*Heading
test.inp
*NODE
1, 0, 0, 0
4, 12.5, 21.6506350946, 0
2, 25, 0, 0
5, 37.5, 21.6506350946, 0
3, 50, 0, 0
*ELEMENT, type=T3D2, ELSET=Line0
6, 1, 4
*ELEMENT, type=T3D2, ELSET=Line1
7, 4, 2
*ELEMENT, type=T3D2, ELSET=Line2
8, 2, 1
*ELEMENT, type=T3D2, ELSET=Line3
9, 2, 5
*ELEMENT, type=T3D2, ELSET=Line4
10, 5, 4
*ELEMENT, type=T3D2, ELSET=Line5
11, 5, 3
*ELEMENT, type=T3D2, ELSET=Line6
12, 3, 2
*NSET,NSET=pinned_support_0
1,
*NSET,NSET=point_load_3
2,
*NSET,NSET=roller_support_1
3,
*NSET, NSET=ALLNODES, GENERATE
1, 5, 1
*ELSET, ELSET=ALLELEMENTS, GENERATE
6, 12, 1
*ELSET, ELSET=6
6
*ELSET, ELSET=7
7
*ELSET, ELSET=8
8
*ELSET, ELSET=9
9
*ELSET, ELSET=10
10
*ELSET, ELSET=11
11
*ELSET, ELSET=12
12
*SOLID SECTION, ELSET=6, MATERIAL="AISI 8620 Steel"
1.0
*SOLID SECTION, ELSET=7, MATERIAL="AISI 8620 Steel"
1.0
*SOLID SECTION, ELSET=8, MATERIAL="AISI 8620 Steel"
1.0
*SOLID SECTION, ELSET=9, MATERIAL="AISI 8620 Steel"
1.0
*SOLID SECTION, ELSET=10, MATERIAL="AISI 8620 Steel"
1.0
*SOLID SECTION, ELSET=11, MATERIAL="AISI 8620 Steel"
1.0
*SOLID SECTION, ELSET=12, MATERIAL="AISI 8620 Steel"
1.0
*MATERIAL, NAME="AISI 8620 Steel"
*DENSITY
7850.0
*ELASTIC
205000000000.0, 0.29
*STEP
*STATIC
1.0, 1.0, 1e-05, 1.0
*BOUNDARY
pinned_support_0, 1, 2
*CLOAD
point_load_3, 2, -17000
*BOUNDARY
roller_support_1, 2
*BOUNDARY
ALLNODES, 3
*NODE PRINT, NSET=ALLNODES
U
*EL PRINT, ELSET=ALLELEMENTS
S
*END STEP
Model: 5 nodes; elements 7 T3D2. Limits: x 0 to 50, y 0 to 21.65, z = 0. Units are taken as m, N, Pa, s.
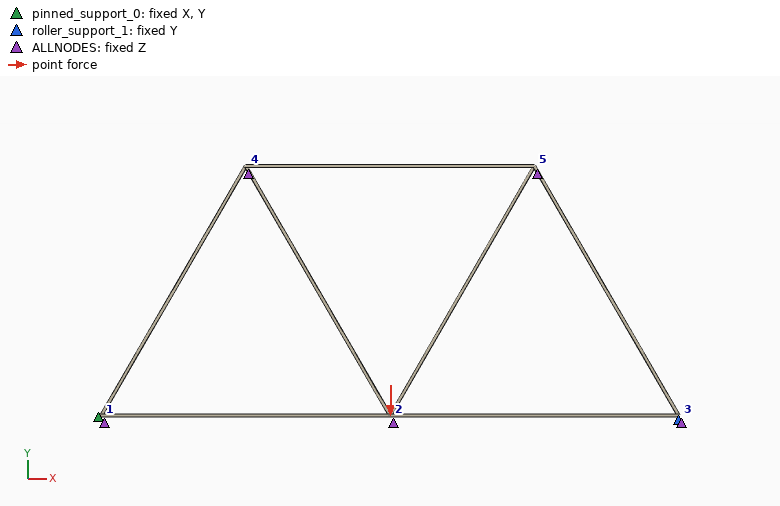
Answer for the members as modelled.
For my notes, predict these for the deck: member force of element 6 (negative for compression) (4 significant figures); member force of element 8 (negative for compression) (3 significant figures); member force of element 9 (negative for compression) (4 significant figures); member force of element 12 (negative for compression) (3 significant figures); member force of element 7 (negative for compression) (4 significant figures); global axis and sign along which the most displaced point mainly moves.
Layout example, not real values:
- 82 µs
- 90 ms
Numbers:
- -9815 N
- 4910 N
- 9815 N
- 4910 N
- 9815 N
- -Y
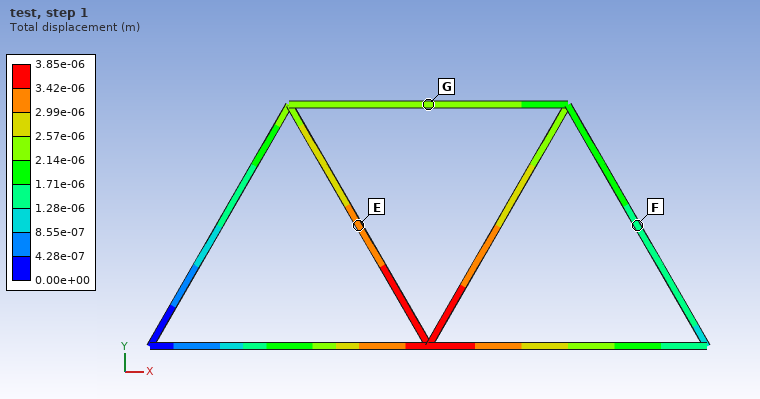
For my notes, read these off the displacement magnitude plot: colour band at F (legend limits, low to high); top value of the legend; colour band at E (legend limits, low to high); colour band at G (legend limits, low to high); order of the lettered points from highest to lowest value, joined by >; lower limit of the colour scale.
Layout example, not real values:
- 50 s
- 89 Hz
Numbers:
- 1.28e-06 to 1.71e-06 m
- 3.85e-06 m
- 2.99e-06 to 3.42e-06 m
- 2.14e-06 to 2.57e-06 m
- E > G > F
- 0.00e+00 m
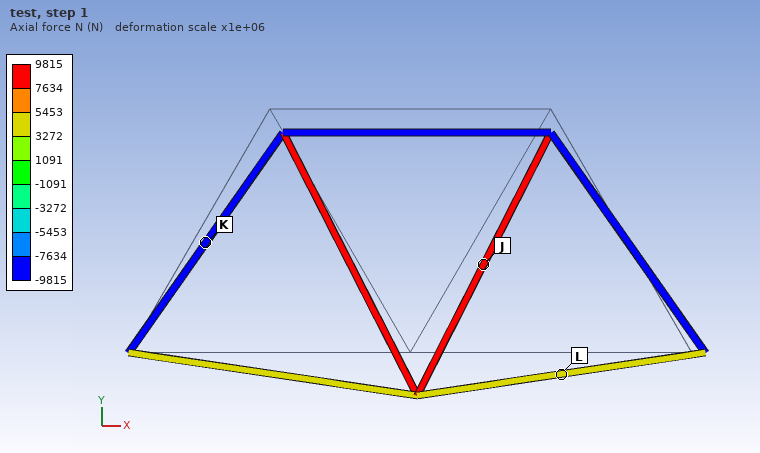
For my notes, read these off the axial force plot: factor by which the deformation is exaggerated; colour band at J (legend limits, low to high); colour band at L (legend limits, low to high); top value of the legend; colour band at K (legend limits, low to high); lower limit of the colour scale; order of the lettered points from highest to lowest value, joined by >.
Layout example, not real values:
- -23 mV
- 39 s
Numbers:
- 1e+06
- 7634 to 9815 N
- 3272 to 5453 N
- 9815 N
- -9815 to -7634 N
- -9815 N
- J > L > K
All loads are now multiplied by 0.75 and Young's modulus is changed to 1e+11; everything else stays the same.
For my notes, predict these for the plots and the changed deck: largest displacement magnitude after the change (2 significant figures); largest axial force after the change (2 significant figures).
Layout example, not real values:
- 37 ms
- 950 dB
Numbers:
- 5.9e-06 m
- 7400 N
